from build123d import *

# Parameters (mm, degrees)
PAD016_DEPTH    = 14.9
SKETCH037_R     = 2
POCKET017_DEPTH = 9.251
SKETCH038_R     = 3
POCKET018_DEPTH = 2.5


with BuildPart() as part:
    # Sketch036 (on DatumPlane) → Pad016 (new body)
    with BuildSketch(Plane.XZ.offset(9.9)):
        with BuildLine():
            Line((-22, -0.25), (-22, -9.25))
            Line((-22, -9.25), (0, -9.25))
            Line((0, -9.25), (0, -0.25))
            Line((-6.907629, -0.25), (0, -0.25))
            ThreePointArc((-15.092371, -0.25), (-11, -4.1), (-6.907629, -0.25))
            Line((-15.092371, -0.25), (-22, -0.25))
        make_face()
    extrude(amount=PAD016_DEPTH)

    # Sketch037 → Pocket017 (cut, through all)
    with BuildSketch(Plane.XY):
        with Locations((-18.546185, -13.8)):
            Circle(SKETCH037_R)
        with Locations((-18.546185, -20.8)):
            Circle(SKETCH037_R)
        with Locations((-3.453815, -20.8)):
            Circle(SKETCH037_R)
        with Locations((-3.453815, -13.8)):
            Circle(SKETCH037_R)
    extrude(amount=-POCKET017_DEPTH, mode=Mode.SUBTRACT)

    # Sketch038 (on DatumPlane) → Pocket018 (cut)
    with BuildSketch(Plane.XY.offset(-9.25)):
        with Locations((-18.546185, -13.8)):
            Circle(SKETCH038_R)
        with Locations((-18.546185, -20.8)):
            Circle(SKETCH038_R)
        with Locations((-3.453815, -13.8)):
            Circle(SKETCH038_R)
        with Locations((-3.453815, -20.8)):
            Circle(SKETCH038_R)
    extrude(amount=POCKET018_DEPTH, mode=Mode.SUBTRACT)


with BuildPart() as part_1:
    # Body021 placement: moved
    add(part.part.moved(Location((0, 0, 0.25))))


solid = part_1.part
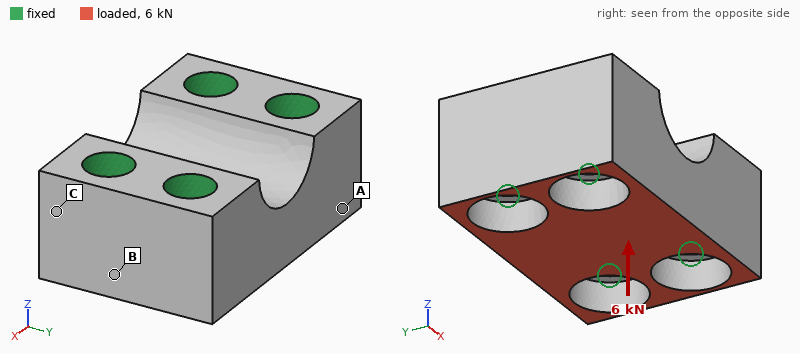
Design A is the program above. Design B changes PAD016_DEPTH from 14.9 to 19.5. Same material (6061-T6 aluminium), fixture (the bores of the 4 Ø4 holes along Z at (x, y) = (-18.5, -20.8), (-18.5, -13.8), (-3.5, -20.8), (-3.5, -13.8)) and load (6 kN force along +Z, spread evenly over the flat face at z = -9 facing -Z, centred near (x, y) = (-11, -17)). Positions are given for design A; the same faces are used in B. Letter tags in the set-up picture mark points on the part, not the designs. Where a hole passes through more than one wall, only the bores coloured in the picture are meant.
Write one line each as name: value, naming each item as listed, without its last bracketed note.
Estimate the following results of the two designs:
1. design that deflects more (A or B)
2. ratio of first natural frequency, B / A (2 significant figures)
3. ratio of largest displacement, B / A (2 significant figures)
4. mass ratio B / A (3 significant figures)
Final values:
design that deflects more: B
ratio of first natural frequency, B / A: 0.60
ratio of largest displacement, B / A: 2.2
mass ratio B / A: 1.40
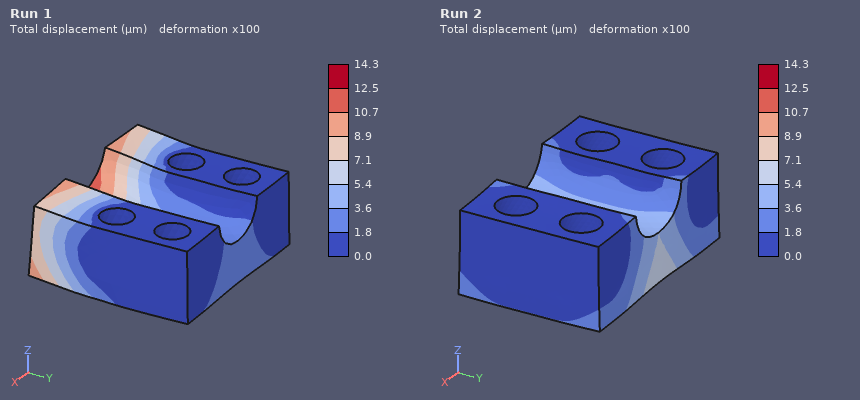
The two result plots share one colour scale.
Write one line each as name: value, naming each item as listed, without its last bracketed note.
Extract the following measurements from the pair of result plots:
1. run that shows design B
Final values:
run that shows design B: Run 1
